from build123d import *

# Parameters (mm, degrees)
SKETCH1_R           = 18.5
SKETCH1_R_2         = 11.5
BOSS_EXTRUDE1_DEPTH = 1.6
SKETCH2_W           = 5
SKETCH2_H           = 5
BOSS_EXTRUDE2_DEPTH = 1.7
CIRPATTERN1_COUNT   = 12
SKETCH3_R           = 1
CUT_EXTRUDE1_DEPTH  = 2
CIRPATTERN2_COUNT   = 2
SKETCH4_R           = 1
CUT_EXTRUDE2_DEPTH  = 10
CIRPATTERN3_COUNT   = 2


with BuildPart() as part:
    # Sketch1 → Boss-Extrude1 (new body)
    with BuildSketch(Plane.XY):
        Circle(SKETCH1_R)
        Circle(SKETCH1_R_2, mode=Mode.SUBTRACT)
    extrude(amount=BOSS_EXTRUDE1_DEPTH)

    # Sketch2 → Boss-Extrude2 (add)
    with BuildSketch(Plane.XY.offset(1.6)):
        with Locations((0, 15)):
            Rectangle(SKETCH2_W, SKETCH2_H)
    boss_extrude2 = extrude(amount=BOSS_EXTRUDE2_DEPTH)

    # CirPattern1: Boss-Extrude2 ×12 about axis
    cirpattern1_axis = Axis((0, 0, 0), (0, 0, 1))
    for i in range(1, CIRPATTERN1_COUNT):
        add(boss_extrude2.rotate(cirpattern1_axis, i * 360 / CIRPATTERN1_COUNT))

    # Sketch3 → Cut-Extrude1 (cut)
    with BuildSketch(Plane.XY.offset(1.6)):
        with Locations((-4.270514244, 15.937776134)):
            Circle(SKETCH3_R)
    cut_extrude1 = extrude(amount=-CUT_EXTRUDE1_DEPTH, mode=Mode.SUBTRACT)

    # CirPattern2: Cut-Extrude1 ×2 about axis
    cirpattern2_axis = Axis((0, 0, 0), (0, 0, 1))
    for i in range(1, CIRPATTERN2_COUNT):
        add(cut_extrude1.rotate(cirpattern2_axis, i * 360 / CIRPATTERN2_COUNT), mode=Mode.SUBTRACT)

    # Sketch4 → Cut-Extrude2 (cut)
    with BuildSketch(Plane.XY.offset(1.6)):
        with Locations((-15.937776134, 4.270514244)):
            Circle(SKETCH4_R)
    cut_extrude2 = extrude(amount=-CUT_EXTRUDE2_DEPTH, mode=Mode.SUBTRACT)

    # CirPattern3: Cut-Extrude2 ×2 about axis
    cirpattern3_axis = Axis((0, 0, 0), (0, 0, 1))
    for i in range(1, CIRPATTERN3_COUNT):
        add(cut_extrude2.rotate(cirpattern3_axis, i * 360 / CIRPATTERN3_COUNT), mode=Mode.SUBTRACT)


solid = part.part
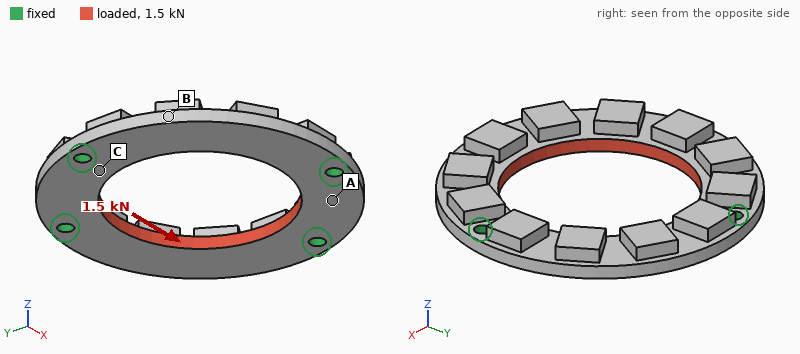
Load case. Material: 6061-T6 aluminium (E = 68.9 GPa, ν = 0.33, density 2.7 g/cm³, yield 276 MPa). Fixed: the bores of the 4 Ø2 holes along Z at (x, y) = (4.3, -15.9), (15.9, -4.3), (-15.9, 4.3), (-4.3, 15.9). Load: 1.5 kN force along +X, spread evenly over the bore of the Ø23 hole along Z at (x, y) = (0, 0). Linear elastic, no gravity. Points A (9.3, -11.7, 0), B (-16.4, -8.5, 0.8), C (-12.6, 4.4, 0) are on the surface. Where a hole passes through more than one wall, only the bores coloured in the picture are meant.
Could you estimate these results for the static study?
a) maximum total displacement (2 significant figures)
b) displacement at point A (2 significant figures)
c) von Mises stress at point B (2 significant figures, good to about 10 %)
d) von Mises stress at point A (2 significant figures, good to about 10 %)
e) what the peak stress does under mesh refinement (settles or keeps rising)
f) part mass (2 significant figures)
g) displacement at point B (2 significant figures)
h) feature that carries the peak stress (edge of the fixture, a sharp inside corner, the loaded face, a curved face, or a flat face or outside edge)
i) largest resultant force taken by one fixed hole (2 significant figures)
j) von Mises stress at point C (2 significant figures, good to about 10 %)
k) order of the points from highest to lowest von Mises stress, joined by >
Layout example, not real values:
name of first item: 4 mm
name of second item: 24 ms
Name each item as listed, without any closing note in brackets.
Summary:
maximum total displacement: 8.9 µm
displacement at point A: 2.8 µm
von Mises stress at point B: 25 MPa
von Mises stress at point A: 9.9 MPa
what the peak stress does under mesh refinement: keeps rising
part mass: 4.2 g
displacement at point B: 7.9 µm
feature that carries the peak stress: edge of the fixture
largest resultant force taken by one fixed hole: 430 N
von Mises stress at point C: 37 MPa
order of the points from highest to lowest von Mises stress, joined by >: C > B > A
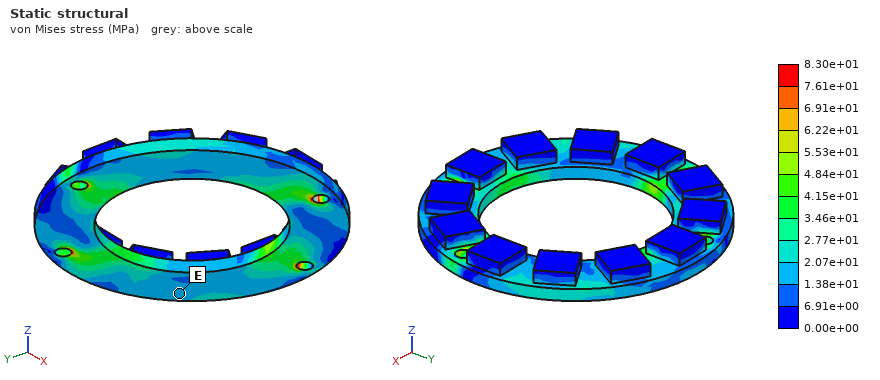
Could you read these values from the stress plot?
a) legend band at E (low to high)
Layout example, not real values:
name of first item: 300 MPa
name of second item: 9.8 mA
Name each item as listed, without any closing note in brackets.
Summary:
legend band at E: 1.38e+01 to 2.07e+01 MPa
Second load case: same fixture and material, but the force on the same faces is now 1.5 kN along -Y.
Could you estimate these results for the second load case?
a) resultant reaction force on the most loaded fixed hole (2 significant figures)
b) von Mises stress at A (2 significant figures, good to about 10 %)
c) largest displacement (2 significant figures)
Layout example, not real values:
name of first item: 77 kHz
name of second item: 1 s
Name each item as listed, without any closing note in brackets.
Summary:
resultant reaction force on the most loaded fixed hole: 430 N
von Mises stress at A: 17 MPa
largest displacement: 8.9 µm
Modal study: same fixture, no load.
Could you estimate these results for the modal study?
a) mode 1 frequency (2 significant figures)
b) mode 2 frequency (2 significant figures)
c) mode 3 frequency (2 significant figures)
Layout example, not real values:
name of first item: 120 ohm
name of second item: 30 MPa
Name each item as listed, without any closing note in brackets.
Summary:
mode 1 frequency: 7300 Hz
mode 2 frequency: 7400 Hz
mode 3 frequency: 20 kHz
